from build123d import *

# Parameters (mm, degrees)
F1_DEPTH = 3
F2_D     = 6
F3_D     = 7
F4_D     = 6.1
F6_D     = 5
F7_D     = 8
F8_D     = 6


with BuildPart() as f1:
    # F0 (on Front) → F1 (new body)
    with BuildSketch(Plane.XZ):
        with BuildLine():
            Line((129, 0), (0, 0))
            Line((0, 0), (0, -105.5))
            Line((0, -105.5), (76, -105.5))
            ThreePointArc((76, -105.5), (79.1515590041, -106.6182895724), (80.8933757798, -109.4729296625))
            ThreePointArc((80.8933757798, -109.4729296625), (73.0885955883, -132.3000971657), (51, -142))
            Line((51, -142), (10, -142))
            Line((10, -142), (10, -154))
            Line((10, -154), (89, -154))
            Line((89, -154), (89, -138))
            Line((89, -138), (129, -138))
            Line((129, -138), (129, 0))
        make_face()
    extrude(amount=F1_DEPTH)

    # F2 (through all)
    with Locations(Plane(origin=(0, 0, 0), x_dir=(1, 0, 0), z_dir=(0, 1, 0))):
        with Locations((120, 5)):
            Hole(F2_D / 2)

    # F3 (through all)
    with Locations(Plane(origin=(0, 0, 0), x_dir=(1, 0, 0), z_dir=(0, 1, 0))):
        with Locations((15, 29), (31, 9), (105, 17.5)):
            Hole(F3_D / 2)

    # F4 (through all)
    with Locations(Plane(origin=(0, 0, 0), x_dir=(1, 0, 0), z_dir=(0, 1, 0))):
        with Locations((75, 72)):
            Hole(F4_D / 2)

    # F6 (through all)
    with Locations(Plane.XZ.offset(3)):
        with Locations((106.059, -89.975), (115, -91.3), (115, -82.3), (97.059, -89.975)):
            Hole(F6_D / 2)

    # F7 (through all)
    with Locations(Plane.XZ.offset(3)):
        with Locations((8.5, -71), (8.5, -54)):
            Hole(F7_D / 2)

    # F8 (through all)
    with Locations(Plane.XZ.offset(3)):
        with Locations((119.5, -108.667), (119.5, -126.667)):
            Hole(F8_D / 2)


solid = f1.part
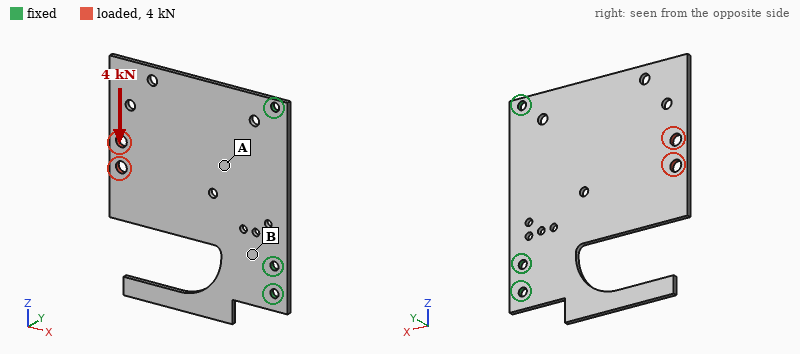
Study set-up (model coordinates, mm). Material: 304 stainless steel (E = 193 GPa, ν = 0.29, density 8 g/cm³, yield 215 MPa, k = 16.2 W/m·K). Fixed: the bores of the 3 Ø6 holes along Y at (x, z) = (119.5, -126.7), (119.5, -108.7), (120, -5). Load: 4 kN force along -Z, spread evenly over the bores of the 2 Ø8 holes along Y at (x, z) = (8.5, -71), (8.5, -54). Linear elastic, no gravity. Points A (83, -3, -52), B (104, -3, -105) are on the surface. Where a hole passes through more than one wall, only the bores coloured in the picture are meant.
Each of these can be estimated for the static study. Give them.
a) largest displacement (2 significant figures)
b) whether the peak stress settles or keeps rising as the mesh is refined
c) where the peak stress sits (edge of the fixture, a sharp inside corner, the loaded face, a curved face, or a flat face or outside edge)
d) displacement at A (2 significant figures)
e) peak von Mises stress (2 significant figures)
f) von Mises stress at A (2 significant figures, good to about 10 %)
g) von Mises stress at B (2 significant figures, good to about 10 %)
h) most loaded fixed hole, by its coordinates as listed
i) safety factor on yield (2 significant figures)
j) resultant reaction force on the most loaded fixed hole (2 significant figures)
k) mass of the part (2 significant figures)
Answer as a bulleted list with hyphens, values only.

- 59 µm
- settles
- a curved face
- 10 µm
- 180 MPa
- 18 MPa
- 52 MPa
- (120, -5)
- 1.2
- 4.2 kN
- 380 g
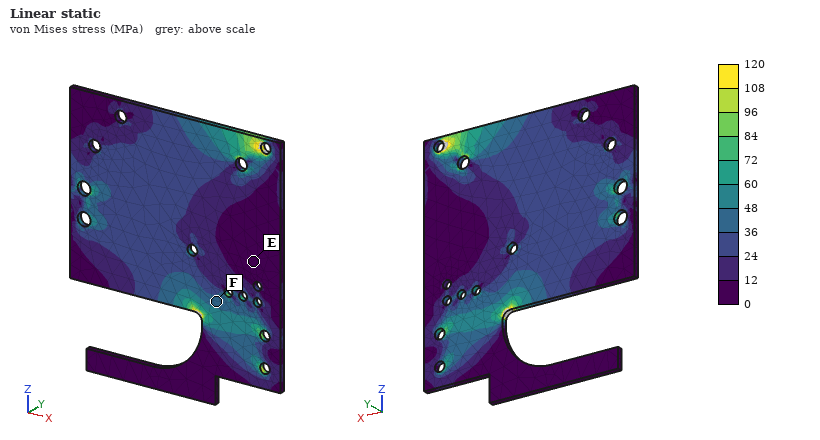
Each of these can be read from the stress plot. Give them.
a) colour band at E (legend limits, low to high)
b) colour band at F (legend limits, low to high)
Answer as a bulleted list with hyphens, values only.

- 0 to 12 MPa
- 36 to 48 MPa
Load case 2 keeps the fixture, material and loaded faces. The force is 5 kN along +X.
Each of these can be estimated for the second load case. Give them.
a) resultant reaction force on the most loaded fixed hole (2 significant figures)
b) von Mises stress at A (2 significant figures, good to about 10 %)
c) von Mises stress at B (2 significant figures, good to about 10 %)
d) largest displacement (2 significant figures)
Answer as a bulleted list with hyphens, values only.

- 2.5 kN
- 9.8 MPa
- 37 MPa
- 22 µm
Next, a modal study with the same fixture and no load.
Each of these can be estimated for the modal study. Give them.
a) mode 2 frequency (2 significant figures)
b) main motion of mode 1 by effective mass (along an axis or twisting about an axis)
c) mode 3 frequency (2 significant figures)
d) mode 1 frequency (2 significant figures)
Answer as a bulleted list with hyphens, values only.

- 300 Hz
- along Y
- 500 Hz
- 150 Hz
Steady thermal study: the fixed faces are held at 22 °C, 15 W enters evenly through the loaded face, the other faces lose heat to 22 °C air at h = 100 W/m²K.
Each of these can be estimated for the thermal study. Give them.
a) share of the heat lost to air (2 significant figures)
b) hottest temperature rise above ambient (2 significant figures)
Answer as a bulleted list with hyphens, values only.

- 100 %
- 81 K
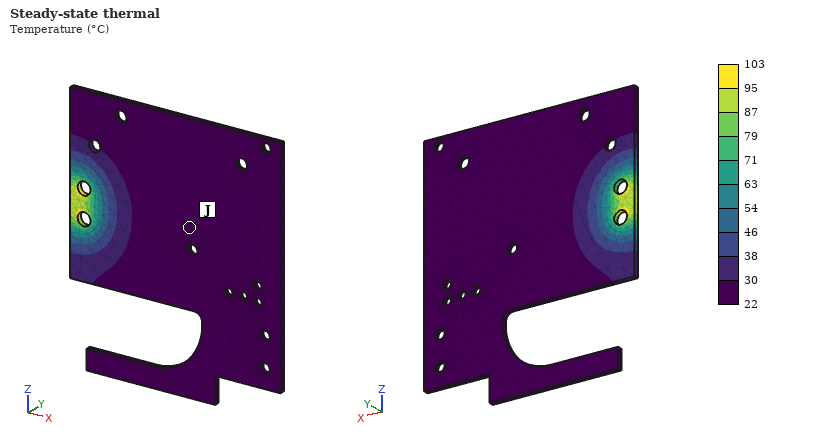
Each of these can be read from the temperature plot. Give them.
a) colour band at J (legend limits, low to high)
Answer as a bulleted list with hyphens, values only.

- 22 to 30 °C
